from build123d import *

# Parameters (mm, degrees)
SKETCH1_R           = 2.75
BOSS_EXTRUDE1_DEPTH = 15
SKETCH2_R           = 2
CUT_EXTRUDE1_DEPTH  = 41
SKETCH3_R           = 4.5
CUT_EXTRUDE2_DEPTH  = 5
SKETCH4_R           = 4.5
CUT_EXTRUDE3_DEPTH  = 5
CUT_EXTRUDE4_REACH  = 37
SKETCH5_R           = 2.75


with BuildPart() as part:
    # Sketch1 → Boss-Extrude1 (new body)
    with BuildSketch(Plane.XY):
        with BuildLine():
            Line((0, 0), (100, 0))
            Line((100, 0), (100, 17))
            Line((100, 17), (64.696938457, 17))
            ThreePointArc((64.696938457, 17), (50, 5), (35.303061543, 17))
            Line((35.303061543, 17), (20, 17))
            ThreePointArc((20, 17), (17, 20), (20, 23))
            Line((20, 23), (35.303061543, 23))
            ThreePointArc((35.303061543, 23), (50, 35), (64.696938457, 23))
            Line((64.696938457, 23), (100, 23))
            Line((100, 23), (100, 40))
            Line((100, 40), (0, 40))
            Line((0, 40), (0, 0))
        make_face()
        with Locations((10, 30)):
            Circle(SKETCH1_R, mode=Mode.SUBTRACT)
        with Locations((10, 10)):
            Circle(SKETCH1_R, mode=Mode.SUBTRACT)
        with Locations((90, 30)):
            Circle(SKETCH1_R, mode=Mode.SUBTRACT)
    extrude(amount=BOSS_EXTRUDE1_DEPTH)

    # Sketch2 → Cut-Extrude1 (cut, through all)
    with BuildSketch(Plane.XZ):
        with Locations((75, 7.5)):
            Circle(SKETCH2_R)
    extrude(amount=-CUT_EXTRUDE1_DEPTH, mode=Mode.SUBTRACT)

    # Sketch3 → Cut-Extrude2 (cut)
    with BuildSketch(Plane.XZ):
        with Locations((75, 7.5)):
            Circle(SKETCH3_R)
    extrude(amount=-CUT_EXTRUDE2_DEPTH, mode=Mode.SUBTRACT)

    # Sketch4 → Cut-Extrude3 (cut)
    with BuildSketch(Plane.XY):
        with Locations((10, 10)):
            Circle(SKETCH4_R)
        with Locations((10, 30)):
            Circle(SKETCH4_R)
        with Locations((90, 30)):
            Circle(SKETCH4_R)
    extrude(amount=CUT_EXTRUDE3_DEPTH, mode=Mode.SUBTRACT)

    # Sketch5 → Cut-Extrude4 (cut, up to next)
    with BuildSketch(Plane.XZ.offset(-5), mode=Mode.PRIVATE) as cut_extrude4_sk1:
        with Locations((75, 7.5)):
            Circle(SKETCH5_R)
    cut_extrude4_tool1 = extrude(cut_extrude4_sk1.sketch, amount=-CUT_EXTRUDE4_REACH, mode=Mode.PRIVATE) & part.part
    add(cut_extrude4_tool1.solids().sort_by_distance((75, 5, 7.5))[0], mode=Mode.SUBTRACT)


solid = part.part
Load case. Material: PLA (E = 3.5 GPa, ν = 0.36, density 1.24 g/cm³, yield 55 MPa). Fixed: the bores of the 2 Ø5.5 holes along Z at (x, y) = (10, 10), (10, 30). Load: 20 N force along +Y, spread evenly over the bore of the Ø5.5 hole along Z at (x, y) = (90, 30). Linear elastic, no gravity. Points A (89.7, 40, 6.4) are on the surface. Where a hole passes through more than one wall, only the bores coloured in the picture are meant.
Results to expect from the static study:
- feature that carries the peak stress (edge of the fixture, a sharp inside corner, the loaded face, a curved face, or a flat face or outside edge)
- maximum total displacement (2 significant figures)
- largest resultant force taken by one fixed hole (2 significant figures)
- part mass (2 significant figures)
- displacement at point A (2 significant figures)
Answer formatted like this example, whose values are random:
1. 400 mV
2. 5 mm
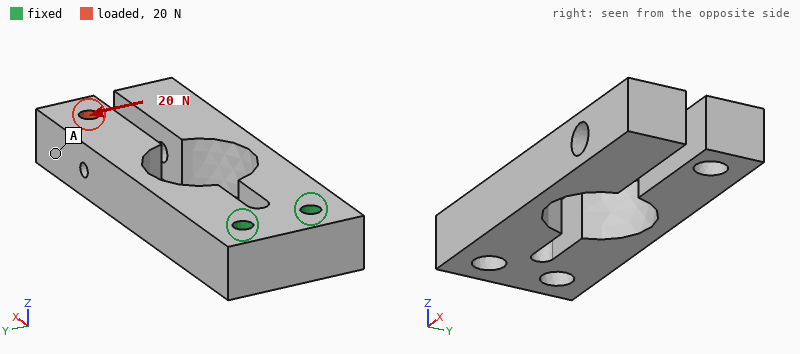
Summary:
1. a flat face or outside edge
2. 1.3 mm
3. 62 N
4. 52 g
5. 1.0 mm
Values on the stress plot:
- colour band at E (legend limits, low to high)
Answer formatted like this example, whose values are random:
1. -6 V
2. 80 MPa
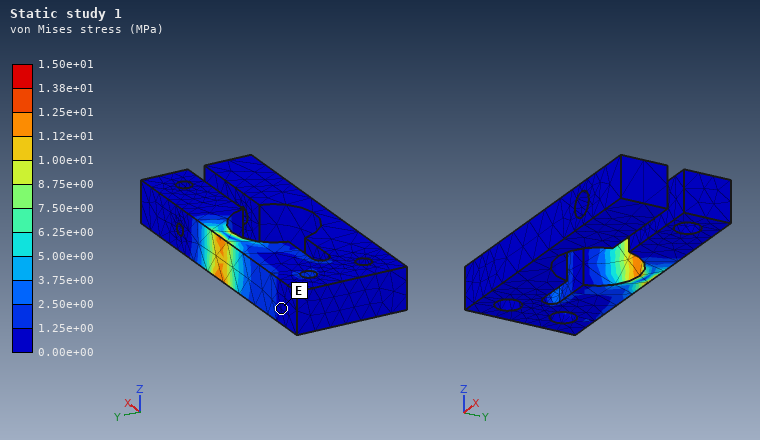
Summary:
1. 0.00e+00 to 1.25e+00 MPa
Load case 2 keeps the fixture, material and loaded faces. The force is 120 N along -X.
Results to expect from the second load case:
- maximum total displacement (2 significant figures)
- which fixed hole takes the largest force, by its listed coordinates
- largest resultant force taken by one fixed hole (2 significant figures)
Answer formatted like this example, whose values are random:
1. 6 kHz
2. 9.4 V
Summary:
1. 1.2 mm
2. (10, 30)
3. 110 N
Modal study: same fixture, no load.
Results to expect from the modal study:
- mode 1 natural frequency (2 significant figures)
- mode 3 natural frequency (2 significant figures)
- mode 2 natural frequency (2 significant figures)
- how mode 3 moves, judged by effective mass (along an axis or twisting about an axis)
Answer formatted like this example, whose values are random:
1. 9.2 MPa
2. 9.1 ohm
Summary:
1. 240 Hz
2. 380 Hz
3. 250 Hz
4. along Z
